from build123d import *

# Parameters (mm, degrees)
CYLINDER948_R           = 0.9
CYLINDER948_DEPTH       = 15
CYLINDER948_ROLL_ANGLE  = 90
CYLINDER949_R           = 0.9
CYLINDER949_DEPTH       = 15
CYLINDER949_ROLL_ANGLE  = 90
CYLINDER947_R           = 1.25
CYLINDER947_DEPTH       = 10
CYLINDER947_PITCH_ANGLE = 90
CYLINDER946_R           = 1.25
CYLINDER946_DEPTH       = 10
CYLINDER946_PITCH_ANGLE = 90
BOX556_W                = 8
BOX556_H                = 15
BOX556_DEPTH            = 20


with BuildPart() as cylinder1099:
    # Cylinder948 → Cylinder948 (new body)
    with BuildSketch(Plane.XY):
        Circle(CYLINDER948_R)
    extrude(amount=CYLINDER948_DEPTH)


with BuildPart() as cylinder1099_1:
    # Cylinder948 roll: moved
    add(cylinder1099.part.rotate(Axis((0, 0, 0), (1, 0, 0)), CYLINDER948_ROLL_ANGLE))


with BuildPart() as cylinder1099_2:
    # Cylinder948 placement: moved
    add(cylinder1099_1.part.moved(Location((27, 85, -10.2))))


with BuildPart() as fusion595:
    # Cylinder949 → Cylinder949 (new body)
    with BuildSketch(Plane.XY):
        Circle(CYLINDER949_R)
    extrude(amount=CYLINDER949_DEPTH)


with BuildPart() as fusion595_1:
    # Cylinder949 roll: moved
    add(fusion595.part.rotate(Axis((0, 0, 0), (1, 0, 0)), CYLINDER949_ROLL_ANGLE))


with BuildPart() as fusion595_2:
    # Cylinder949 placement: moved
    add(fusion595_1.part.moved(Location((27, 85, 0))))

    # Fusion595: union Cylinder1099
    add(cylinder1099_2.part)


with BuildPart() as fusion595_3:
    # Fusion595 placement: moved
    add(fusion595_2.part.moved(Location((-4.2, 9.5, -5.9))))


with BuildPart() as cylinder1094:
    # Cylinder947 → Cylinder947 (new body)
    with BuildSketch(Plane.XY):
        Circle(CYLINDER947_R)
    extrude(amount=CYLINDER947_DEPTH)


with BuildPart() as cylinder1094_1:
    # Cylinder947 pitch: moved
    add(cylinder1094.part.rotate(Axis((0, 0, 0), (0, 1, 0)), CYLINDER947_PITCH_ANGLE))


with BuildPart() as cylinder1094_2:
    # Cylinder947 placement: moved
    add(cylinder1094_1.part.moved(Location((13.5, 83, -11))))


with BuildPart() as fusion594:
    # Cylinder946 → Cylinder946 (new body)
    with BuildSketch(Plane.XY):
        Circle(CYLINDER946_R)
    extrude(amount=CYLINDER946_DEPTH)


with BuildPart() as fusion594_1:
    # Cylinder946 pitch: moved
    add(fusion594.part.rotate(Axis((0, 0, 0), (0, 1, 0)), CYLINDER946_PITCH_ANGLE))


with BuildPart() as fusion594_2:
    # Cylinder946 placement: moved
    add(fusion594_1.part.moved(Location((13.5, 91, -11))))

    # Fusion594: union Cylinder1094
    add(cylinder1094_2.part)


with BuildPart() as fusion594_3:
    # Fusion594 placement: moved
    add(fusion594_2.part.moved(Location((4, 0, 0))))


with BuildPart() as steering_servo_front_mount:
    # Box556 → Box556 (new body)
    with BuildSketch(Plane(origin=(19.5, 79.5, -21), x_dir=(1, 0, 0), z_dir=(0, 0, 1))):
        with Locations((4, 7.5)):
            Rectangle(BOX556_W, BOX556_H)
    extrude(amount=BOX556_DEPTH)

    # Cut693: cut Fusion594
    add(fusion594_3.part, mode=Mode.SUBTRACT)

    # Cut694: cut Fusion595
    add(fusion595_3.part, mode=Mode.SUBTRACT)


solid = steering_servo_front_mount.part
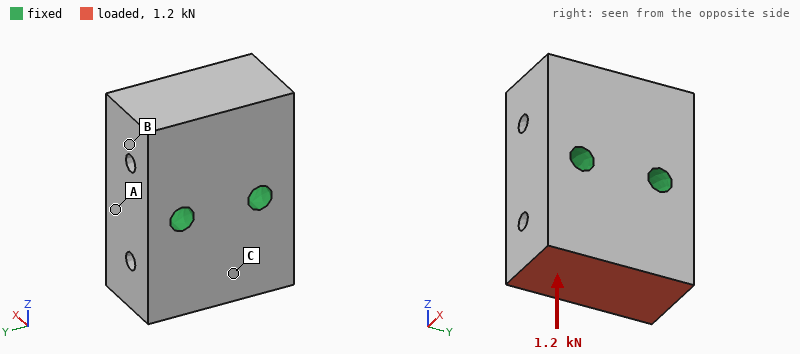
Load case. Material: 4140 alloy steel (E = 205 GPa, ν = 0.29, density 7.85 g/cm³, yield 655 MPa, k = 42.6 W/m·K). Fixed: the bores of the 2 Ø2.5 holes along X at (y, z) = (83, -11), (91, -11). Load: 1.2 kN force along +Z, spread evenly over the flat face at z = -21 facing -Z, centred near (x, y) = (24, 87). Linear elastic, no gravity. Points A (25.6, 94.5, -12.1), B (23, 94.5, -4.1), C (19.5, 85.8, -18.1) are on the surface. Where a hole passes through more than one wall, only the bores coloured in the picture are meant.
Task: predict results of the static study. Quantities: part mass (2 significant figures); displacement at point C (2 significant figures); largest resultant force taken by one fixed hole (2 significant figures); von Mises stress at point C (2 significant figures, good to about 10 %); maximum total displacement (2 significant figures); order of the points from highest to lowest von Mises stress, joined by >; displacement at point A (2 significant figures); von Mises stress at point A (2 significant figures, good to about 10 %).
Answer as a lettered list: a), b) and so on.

a) 18 g
b) 0.39 µm
c) 600 N
d) 11 MPa
e) 0.59 µm
f) C > A > B
g) 0.15 µm
h) 6.0 MPa
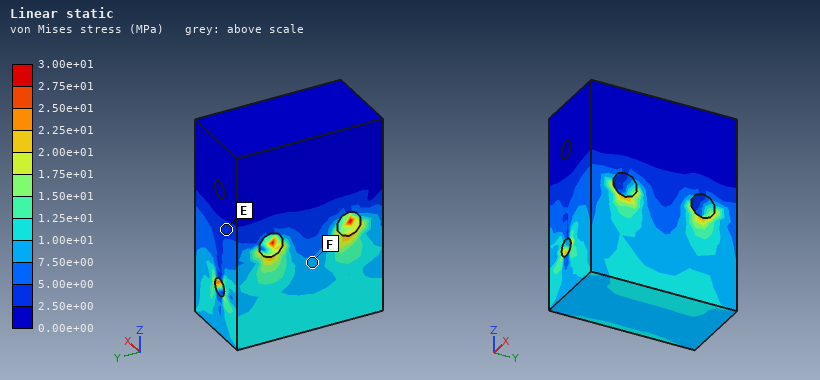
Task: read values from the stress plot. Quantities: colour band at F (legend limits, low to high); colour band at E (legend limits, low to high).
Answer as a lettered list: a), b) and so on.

a) 7.50e+00 to 1.00e+01 MPa
b) 2.50e+00 to 5.00e+00 MPa
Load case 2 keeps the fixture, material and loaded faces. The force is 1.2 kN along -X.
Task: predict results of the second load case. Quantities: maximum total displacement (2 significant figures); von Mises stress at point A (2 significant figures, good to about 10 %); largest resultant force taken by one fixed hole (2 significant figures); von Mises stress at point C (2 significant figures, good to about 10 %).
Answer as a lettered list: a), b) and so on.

a) 5.2 µm
b) 15 MPa
c) 600 N
d) 18 MPa
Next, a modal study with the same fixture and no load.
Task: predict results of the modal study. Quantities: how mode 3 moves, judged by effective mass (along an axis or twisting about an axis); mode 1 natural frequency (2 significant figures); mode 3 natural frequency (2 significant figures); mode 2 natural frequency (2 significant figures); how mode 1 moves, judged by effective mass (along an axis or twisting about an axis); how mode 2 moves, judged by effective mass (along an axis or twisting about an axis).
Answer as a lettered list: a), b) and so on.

a) twisting about X
b) 45 kHz
c) 55 kHz
d) 51 kHz
e) twisting about Y
f) along X
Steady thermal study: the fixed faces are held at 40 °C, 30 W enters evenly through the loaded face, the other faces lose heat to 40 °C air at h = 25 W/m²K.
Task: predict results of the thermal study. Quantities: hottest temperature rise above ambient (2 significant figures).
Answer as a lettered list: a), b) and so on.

a) 60 K
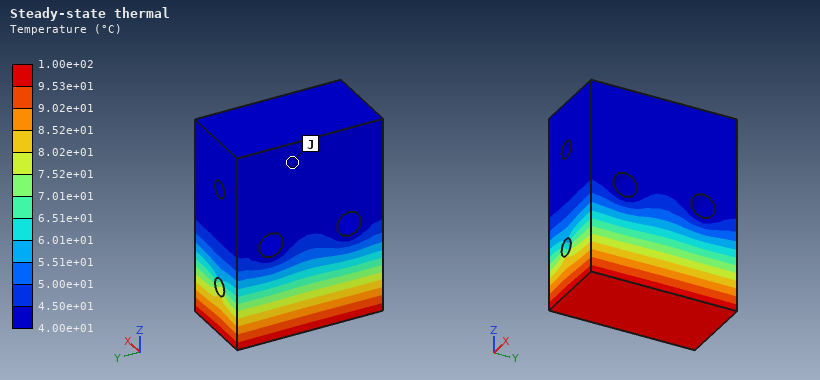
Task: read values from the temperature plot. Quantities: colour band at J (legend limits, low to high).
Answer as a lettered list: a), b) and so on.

a) 4.00e+01 to 4.50e+01 °C
